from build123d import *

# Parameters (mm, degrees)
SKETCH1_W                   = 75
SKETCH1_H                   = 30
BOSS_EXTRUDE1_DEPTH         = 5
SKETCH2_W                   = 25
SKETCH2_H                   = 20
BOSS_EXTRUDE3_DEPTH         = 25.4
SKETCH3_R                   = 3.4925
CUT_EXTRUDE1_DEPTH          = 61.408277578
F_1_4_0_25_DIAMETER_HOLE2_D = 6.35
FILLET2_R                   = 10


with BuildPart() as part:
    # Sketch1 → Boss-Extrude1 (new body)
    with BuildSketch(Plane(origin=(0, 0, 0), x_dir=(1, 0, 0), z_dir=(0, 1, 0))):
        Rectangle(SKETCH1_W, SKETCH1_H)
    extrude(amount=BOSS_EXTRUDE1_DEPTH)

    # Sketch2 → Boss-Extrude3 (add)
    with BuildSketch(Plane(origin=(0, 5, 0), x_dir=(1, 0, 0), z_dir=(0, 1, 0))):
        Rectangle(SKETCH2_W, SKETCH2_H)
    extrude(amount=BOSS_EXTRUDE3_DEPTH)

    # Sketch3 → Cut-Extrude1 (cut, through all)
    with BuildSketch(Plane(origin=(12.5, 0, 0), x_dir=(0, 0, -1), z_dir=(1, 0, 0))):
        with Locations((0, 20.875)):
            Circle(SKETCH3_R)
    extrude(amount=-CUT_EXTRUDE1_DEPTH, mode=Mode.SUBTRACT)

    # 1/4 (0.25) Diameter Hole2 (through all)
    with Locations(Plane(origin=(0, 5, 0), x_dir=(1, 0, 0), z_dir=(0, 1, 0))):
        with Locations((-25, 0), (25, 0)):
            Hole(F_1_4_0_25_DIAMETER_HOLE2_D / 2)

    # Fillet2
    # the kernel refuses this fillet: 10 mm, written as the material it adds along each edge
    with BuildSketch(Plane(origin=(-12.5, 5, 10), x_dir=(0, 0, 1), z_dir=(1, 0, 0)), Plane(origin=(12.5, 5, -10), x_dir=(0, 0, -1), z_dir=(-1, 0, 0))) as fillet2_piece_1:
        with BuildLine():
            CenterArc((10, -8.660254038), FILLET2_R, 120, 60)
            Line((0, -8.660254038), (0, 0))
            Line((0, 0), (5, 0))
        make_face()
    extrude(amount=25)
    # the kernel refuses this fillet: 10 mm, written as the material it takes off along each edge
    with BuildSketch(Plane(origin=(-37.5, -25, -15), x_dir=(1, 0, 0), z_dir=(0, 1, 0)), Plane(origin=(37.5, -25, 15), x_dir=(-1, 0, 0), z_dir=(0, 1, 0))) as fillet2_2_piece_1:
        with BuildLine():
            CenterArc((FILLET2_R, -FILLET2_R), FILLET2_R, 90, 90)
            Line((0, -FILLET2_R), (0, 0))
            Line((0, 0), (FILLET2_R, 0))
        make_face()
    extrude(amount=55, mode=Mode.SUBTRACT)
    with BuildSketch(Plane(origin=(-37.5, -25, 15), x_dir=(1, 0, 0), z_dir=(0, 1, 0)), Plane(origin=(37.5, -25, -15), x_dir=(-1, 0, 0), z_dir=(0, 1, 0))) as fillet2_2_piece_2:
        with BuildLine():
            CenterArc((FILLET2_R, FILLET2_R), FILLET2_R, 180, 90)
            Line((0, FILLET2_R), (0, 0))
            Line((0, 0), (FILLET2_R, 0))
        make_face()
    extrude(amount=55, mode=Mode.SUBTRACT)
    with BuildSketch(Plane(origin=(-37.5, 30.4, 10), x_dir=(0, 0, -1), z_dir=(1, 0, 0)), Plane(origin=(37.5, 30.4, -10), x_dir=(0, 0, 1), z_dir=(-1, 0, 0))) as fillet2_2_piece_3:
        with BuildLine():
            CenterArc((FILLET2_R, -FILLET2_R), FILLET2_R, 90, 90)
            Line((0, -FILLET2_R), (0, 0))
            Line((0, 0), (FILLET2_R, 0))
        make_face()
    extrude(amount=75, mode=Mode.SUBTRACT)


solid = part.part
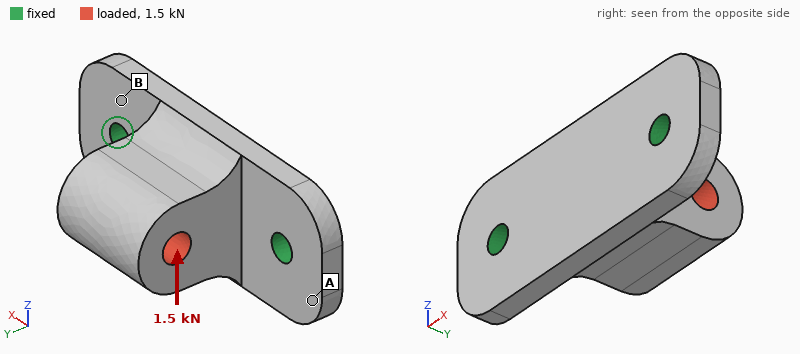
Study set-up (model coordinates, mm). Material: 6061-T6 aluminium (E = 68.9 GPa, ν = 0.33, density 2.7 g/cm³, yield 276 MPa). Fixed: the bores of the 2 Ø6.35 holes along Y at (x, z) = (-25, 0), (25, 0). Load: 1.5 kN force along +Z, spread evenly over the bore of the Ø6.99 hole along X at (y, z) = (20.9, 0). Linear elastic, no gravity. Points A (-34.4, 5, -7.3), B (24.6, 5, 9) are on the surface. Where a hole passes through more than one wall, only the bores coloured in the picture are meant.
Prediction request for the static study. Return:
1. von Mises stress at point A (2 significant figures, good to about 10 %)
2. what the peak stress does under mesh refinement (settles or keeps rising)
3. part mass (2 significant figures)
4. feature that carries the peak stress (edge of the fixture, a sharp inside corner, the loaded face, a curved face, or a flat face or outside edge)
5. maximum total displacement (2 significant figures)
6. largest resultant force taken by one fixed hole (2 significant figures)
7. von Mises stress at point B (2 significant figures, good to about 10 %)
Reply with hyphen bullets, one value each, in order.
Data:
- 22 MPa
- keeps rising
- 59 g
- edge of the fixture
- 0.13 mm
- 750 N
- 47 MPa
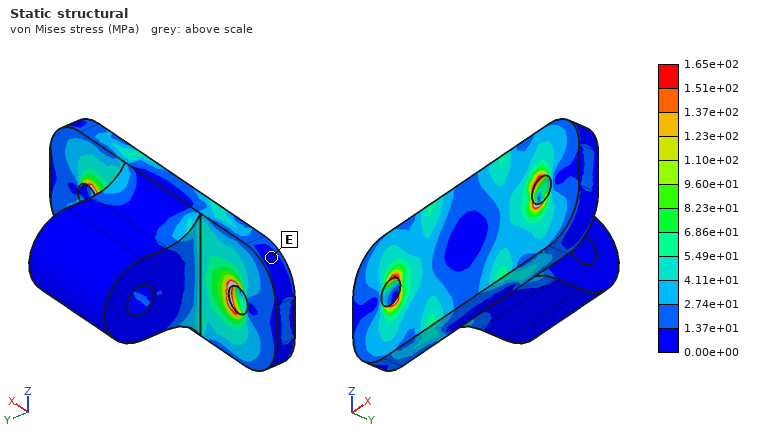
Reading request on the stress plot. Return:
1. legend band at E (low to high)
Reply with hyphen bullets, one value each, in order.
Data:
- 0.00e+00 to 1.37e+01 MPa
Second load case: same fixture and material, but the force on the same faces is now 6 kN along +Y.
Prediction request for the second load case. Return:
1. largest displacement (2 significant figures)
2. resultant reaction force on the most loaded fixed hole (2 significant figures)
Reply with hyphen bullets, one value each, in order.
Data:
- 61 µm
- 3.3 kN
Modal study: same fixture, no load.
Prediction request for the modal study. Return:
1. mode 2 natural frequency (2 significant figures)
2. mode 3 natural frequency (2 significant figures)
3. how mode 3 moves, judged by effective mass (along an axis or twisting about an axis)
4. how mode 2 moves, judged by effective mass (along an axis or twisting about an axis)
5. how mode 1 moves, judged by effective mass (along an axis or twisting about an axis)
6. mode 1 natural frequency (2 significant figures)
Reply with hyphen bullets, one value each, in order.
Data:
- 7800 Hz
- 9200 Hz
- along X
- along Y
- along Z
- 4000 Hz
